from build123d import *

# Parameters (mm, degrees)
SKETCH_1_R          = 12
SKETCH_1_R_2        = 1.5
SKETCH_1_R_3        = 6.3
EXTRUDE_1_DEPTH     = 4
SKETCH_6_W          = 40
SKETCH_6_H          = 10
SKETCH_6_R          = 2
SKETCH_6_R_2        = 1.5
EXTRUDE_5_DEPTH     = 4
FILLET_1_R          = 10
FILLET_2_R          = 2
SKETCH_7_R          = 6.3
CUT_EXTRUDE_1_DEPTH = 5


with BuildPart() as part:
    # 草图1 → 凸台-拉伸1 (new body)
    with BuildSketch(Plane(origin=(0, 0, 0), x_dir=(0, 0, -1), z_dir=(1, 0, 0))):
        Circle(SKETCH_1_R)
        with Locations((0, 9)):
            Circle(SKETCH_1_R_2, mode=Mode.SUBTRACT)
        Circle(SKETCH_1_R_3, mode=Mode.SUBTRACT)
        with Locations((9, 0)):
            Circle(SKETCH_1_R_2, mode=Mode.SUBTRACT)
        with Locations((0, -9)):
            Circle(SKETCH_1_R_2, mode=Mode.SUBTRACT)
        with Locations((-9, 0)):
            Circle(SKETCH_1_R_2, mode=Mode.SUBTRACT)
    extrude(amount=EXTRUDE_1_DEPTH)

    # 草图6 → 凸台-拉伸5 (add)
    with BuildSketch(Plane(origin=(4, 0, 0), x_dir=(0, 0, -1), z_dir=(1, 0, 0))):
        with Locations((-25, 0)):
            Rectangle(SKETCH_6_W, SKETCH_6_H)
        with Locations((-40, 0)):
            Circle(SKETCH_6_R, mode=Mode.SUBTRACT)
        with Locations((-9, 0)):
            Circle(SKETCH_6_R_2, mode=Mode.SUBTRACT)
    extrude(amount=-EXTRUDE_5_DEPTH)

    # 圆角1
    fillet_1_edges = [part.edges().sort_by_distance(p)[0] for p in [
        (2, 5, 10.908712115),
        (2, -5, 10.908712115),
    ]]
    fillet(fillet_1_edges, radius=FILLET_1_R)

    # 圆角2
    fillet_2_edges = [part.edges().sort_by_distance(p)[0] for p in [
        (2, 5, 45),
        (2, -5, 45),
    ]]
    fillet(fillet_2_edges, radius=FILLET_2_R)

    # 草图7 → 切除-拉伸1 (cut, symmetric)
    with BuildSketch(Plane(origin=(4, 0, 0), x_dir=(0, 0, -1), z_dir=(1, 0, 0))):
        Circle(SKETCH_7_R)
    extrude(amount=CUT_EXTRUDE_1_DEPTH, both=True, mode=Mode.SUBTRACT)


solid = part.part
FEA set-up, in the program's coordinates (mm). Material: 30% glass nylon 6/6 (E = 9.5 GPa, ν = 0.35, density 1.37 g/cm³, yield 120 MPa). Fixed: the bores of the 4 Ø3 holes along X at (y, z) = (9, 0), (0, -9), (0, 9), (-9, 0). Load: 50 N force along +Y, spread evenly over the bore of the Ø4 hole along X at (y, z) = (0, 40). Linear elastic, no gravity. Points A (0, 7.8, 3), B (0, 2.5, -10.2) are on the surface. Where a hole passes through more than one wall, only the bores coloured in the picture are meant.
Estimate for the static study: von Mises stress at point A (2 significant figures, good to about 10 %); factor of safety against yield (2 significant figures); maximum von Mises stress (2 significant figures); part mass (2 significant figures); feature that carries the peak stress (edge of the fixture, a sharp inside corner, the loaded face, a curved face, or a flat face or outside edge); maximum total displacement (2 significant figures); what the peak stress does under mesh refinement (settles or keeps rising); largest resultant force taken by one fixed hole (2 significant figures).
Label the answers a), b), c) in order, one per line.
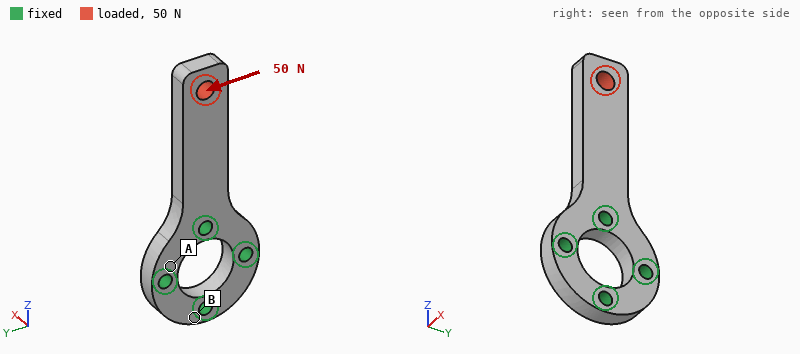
a) 4.6 MPa
b) 5.6
c) 21 MPa
d) 3.4 g
e) a curved face
f) 0.20 mm
g) settles
h) 86 N
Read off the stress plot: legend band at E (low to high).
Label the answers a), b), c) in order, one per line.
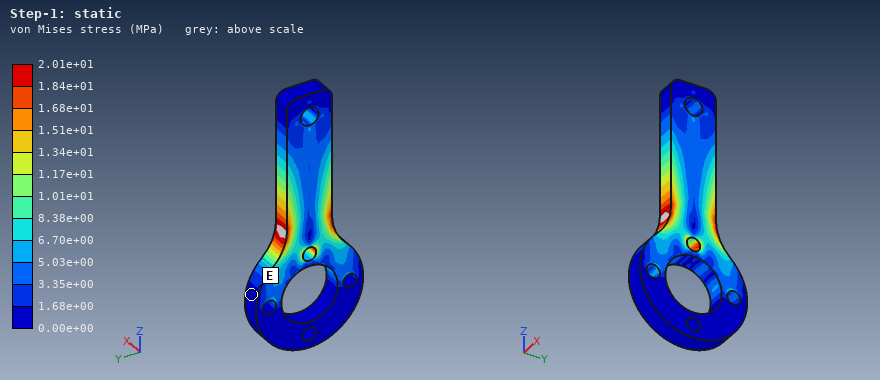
a) 0.00e+00 to 1.68e+00 MPa
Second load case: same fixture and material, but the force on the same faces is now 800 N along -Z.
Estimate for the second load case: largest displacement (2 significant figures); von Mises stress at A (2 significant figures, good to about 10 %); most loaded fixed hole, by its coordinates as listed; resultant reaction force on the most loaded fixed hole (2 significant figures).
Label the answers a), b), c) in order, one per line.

a) 81 µm
b) 5.0 MPa
c) (0, 9)
d) 620 N
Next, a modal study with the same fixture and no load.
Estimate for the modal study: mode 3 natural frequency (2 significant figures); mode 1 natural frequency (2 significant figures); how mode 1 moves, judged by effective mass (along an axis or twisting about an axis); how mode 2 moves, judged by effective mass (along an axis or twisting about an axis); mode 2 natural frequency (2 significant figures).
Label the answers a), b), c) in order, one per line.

a) 7600 Hz
b) 1500 Hz
c) along X
d) along Y
e) 3300 Hz
